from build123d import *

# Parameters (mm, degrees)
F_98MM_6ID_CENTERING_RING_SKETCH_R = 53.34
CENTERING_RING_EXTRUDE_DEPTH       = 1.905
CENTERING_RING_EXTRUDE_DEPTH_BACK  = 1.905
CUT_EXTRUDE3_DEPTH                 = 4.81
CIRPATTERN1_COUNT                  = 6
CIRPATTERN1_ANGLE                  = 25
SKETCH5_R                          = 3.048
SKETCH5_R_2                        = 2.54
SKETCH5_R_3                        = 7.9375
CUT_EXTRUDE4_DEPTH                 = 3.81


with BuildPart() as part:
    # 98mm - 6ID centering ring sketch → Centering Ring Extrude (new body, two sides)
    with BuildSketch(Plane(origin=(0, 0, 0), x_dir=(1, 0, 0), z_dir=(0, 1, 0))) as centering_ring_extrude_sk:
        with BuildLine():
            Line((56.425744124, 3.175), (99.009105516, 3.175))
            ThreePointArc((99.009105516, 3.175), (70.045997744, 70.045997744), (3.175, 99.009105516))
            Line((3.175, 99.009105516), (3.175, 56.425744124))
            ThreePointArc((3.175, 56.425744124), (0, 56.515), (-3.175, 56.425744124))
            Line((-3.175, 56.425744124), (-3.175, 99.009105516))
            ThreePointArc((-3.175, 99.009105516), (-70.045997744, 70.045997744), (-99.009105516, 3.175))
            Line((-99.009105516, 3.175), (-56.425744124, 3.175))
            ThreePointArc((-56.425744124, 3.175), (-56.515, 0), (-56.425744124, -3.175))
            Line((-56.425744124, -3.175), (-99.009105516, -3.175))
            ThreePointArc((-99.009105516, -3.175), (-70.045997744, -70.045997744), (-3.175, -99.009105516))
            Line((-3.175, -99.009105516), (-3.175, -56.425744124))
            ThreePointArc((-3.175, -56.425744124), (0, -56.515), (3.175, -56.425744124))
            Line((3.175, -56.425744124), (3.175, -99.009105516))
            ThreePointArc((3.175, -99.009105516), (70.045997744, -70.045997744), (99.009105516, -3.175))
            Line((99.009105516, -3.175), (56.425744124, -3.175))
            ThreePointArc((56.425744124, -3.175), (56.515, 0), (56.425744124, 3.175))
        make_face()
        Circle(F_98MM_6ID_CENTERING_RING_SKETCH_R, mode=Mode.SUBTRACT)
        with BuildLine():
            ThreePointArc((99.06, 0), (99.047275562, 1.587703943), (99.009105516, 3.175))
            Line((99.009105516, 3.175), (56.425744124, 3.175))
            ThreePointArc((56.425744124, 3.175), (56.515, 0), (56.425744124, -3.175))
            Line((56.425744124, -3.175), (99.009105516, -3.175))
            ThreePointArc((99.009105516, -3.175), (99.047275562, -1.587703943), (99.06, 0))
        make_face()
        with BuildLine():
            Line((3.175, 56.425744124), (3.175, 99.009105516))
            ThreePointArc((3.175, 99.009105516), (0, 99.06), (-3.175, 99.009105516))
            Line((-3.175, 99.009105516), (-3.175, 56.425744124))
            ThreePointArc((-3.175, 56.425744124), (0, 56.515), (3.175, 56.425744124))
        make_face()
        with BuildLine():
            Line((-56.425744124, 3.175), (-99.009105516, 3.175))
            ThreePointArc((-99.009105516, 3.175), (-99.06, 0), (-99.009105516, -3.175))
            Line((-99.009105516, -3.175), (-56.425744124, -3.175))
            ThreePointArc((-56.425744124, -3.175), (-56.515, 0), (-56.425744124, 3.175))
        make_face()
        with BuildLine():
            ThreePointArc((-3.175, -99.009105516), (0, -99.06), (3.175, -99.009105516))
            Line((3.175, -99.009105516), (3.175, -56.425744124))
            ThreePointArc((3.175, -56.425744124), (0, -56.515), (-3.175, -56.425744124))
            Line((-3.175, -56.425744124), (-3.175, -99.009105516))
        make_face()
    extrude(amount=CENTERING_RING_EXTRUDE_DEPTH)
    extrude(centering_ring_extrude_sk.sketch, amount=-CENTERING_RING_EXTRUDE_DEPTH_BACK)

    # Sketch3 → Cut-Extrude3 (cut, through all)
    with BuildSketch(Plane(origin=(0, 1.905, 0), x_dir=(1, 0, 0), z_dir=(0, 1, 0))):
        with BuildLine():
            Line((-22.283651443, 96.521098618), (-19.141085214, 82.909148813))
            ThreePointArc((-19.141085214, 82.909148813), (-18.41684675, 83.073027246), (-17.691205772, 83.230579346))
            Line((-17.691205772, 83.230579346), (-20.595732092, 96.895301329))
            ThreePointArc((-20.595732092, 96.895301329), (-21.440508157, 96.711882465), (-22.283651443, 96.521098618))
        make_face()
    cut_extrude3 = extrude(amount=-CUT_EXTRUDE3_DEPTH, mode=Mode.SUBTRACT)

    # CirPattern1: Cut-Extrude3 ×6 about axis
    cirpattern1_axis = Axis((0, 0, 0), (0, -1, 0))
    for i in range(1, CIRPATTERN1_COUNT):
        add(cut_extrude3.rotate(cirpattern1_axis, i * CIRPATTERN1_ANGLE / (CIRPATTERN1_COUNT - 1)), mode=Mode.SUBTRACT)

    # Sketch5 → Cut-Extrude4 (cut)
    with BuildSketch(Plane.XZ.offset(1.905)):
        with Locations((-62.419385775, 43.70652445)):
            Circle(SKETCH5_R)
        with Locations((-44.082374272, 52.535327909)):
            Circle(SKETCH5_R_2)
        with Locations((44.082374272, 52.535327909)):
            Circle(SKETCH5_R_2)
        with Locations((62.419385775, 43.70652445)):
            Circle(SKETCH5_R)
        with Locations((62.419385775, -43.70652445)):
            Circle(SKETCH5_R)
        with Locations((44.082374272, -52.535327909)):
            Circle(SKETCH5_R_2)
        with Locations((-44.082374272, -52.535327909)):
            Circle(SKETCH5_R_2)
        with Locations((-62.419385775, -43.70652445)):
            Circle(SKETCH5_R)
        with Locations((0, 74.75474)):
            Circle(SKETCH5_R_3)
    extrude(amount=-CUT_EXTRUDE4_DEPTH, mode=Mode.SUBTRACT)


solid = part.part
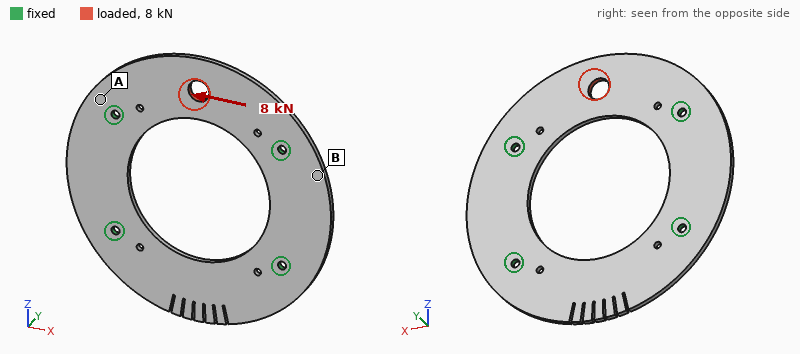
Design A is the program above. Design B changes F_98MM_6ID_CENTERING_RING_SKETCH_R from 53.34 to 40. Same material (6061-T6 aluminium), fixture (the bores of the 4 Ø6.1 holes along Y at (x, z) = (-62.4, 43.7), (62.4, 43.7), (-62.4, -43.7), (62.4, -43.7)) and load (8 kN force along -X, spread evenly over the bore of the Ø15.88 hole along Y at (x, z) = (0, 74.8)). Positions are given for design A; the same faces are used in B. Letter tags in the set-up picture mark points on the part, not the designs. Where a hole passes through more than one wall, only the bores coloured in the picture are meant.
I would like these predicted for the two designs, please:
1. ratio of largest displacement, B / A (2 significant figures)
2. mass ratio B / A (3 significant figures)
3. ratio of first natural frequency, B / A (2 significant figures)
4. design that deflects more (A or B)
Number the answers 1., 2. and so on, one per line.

1. 0.84
2. 1.18
3. 1.1
4. A
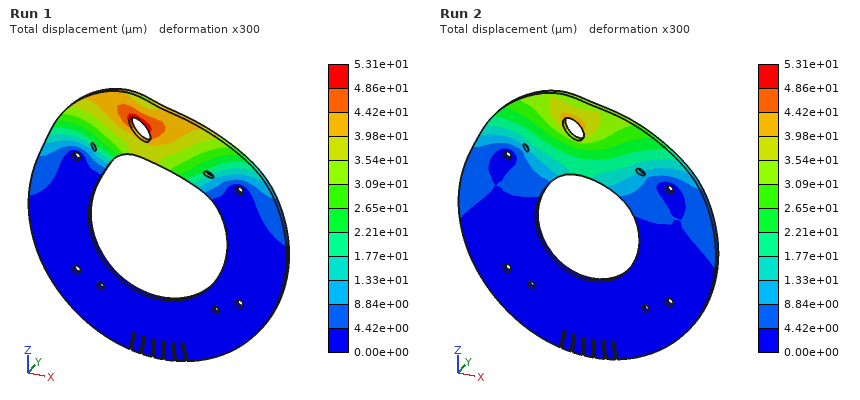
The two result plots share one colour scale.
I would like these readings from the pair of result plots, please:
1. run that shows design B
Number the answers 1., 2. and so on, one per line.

1. Run 2
